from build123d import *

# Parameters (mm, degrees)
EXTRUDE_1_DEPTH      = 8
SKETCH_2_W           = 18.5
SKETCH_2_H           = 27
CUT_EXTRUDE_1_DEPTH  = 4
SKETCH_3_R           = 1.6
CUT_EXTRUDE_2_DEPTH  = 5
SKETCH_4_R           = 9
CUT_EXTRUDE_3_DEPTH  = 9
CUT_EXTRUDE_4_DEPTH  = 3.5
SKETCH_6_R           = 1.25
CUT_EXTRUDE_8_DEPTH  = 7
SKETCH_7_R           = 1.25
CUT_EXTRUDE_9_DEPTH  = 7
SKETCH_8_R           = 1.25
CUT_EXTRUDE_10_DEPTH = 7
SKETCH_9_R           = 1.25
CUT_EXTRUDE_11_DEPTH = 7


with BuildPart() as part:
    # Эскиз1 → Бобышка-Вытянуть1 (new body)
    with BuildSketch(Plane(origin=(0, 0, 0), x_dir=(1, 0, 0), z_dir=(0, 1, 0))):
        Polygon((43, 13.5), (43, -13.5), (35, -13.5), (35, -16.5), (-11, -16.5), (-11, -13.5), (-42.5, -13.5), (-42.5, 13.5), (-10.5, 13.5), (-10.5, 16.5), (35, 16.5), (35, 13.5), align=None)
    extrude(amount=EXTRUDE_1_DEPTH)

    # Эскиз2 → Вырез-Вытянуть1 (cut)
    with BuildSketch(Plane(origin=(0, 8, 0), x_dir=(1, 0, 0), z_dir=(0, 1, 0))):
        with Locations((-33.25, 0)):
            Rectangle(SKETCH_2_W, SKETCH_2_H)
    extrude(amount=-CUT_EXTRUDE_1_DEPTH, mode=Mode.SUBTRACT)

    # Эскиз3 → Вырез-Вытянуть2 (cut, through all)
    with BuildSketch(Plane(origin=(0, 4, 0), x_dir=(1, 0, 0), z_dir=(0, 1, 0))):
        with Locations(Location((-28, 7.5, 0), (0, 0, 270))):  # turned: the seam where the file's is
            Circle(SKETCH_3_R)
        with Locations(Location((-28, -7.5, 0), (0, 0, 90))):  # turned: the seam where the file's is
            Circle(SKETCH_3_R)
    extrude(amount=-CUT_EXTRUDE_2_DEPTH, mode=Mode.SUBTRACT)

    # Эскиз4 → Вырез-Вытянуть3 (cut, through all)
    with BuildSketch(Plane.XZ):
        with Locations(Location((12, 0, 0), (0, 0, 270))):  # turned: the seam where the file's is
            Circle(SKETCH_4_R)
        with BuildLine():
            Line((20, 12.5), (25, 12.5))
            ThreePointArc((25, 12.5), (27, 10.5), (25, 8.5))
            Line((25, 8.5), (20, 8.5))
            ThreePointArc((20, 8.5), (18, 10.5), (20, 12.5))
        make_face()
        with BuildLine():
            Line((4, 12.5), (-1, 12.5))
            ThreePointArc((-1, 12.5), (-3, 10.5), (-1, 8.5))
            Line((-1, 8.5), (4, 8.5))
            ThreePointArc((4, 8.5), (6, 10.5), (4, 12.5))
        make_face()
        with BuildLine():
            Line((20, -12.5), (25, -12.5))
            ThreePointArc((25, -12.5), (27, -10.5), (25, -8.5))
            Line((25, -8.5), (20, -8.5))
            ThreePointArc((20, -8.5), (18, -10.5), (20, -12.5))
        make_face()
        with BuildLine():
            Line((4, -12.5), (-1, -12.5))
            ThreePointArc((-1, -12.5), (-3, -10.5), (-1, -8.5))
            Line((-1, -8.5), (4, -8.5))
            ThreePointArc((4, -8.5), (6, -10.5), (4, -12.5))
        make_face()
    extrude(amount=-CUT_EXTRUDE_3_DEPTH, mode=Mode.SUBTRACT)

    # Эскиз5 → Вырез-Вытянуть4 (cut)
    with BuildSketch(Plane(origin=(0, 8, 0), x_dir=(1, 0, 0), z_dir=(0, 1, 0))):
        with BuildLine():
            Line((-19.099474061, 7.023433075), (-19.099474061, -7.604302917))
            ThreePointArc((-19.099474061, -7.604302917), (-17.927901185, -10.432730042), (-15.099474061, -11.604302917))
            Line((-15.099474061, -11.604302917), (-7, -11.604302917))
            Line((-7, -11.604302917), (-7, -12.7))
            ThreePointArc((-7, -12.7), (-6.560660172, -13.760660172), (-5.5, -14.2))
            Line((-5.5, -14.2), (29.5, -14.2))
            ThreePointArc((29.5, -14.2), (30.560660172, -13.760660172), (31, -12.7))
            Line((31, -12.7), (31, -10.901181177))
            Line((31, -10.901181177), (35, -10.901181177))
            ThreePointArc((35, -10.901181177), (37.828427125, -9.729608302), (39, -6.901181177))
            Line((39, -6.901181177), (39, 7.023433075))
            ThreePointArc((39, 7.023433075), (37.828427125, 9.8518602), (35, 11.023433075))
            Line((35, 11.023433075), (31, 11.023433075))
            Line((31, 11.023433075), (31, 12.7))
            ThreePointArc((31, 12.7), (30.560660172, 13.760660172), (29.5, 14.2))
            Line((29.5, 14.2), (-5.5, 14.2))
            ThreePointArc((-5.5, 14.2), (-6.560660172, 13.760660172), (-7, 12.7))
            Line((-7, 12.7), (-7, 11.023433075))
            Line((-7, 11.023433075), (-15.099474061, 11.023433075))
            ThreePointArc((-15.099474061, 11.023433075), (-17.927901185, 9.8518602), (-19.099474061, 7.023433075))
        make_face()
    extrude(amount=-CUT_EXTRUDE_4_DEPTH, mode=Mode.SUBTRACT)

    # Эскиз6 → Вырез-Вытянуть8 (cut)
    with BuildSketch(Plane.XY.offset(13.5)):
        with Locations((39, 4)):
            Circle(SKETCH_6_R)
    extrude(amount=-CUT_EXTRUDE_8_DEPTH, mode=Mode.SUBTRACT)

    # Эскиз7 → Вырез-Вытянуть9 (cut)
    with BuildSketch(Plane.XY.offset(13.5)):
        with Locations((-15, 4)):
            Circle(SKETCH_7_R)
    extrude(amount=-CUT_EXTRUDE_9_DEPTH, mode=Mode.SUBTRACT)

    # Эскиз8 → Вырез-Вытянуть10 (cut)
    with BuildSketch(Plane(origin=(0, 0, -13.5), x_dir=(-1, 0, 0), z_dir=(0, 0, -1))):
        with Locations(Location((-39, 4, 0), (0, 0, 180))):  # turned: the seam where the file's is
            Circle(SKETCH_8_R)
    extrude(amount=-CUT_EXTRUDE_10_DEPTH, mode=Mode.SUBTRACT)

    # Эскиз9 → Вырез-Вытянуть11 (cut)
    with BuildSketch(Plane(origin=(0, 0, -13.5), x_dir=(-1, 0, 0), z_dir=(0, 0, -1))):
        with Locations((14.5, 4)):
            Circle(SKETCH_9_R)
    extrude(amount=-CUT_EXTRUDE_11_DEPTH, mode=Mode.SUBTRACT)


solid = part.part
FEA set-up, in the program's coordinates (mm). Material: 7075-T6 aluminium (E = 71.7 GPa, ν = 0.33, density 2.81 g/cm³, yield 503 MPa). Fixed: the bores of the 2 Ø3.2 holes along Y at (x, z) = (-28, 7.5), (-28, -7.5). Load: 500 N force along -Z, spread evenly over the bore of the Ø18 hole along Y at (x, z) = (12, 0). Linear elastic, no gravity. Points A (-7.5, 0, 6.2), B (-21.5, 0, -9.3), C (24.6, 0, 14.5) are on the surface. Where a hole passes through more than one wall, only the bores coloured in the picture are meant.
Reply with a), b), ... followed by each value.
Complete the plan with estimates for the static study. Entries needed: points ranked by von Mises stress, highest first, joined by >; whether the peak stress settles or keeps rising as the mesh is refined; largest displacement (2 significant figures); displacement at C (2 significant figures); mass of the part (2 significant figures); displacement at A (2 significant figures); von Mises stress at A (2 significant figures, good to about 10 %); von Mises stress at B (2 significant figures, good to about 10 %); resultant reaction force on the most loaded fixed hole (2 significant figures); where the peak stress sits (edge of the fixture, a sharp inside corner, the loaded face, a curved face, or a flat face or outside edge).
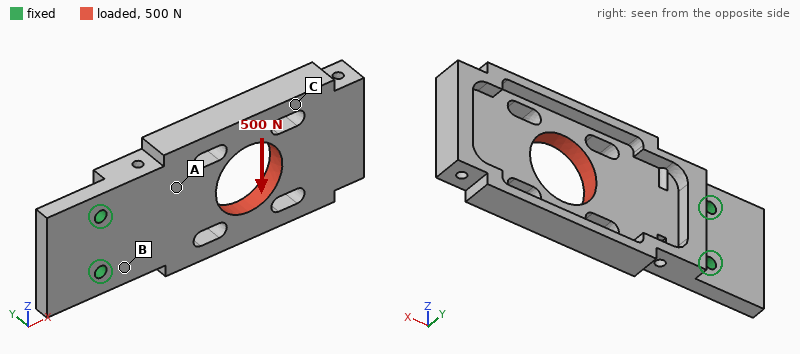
a) B > A > C
b) keeps rising
c) 67 µm
d) 50 µm
e) 32 g
f) 14 µm
g) 12 MPa
h) 27 MPa
i) 1.2 kN
j) edge of the fixture
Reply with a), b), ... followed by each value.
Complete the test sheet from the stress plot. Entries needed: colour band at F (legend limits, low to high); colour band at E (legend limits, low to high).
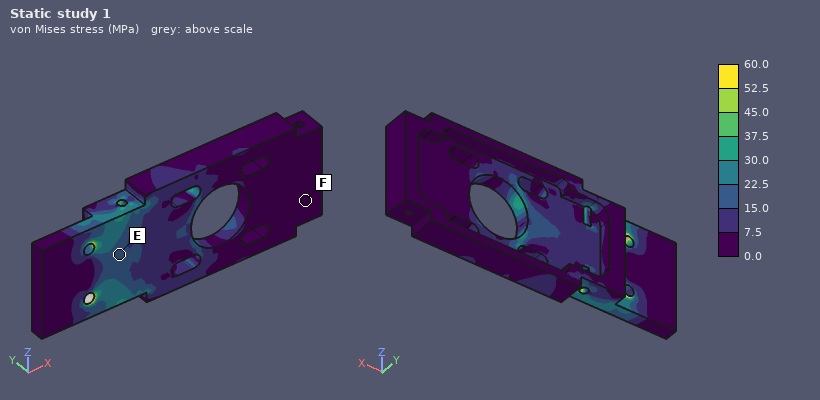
a) 0.0 to 7.5 MPa
b) 15.0 to 22.5 MPa
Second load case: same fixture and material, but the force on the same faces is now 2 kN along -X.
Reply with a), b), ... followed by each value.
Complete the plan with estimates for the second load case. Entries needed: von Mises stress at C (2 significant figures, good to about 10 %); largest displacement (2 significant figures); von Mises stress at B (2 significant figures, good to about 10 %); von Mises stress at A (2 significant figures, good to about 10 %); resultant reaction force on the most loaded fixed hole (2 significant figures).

a) 14 MPa
b) 50 µm
c) 22 MPa
d) 20 MPa
e) 1.0 kN
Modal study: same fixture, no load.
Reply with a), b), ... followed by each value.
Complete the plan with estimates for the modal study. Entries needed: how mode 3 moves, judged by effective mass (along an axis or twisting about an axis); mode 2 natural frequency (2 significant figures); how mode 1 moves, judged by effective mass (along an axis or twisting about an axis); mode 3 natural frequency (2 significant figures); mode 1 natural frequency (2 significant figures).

a) along Z
b) 2600 Hz
c) along Y
d) 3200 Hz
e) 750 Hz
